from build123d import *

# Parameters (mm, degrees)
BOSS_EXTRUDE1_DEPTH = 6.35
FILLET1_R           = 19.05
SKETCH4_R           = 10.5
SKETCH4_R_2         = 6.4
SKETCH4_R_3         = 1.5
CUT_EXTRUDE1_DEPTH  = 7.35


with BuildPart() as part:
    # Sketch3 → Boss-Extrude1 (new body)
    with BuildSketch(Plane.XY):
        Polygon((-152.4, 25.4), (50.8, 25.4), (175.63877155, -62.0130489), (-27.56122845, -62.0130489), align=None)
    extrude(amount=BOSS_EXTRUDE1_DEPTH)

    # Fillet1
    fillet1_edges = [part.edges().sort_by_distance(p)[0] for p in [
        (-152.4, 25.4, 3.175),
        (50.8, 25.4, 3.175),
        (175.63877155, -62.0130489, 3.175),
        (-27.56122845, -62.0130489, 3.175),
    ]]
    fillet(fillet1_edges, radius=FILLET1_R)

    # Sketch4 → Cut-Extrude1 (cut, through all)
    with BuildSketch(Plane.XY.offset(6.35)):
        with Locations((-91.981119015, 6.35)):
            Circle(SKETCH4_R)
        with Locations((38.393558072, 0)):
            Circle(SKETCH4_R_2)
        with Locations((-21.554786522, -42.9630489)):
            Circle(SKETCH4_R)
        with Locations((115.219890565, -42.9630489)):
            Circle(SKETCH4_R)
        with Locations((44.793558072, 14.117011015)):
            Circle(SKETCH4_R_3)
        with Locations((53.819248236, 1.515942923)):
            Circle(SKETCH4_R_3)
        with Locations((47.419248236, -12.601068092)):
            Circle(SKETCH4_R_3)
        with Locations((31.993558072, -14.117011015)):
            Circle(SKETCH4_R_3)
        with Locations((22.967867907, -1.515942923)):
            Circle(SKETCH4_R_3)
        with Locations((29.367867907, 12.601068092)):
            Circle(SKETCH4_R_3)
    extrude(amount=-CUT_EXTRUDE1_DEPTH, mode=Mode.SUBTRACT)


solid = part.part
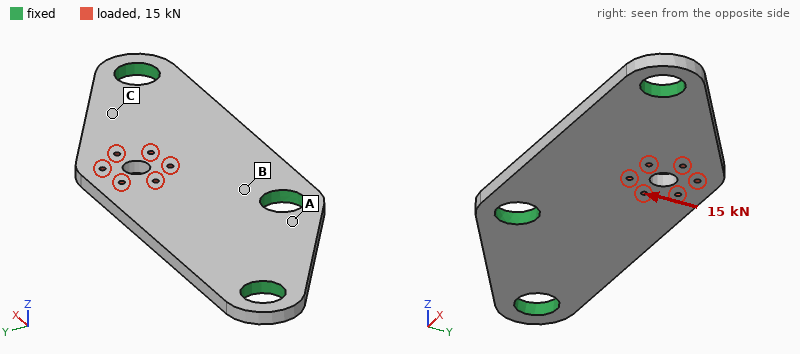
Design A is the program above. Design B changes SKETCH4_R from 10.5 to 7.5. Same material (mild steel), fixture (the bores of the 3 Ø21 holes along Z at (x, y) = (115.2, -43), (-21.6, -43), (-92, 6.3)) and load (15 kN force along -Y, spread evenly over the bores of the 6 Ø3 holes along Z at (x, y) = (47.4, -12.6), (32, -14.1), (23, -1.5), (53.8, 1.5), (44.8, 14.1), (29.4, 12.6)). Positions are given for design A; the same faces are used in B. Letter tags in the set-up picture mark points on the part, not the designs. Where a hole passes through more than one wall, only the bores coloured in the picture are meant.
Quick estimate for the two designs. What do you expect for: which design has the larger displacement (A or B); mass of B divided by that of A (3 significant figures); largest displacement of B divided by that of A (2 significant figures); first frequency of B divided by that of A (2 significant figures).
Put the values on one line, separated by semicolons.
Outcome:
B; 1.03; 1.1; 0.91
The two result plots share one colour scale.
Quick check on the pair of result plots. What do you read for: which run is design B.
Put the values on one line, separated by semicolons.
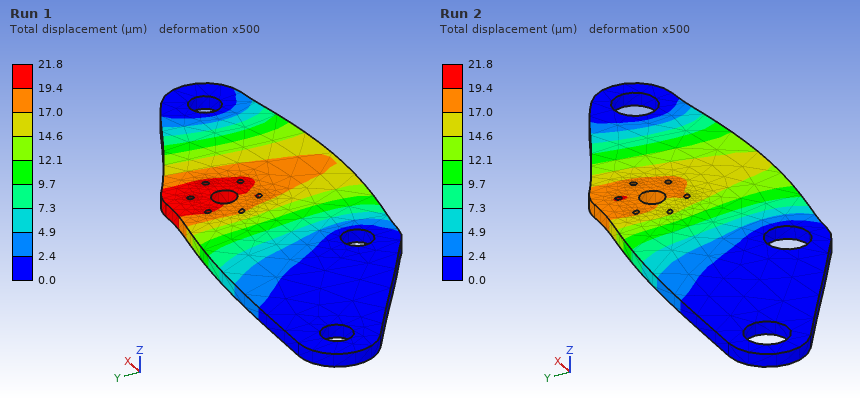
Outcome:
Run 1
